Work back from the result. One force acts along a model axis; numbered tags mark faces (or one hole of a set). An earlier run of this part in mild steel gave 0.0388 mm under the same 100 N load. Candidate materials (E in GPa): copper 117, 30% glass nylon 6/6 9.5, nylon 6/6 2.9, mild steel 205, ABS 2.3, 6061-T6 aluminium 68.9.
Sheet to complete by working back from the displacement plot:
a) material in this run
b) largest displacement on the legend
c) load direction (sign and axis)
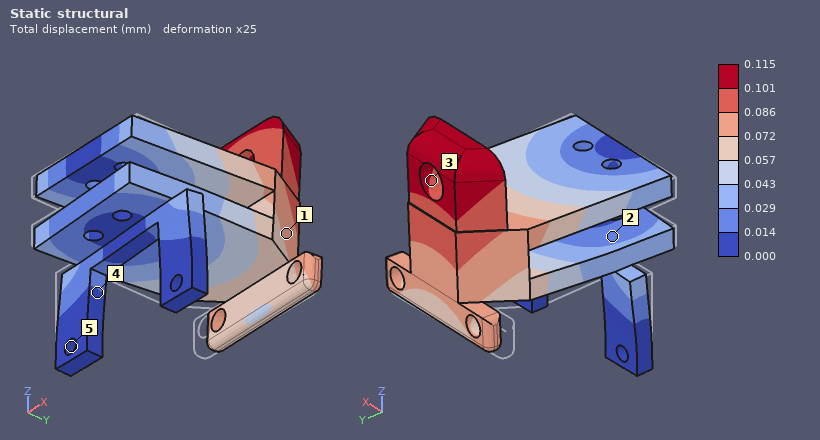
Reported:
6061-T6 aluminium
0.115 mm
+X
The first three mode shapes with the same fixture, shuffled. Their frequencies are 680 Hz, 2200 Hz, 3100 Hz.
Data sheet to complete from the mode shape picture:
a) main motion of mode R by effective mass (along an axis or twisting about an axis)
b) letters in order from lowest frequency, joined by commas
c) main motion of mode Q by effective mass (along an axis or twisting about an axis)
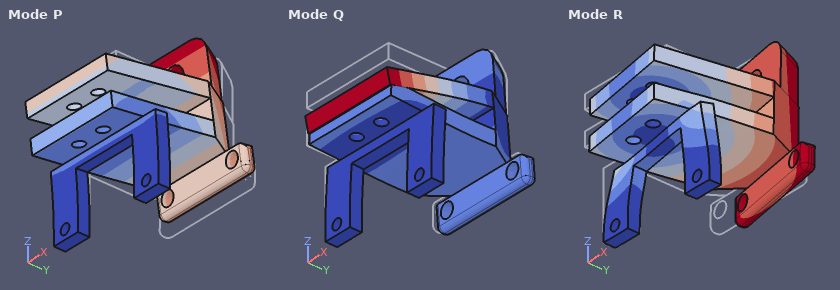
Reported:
along X
P, R, Q
along Z
